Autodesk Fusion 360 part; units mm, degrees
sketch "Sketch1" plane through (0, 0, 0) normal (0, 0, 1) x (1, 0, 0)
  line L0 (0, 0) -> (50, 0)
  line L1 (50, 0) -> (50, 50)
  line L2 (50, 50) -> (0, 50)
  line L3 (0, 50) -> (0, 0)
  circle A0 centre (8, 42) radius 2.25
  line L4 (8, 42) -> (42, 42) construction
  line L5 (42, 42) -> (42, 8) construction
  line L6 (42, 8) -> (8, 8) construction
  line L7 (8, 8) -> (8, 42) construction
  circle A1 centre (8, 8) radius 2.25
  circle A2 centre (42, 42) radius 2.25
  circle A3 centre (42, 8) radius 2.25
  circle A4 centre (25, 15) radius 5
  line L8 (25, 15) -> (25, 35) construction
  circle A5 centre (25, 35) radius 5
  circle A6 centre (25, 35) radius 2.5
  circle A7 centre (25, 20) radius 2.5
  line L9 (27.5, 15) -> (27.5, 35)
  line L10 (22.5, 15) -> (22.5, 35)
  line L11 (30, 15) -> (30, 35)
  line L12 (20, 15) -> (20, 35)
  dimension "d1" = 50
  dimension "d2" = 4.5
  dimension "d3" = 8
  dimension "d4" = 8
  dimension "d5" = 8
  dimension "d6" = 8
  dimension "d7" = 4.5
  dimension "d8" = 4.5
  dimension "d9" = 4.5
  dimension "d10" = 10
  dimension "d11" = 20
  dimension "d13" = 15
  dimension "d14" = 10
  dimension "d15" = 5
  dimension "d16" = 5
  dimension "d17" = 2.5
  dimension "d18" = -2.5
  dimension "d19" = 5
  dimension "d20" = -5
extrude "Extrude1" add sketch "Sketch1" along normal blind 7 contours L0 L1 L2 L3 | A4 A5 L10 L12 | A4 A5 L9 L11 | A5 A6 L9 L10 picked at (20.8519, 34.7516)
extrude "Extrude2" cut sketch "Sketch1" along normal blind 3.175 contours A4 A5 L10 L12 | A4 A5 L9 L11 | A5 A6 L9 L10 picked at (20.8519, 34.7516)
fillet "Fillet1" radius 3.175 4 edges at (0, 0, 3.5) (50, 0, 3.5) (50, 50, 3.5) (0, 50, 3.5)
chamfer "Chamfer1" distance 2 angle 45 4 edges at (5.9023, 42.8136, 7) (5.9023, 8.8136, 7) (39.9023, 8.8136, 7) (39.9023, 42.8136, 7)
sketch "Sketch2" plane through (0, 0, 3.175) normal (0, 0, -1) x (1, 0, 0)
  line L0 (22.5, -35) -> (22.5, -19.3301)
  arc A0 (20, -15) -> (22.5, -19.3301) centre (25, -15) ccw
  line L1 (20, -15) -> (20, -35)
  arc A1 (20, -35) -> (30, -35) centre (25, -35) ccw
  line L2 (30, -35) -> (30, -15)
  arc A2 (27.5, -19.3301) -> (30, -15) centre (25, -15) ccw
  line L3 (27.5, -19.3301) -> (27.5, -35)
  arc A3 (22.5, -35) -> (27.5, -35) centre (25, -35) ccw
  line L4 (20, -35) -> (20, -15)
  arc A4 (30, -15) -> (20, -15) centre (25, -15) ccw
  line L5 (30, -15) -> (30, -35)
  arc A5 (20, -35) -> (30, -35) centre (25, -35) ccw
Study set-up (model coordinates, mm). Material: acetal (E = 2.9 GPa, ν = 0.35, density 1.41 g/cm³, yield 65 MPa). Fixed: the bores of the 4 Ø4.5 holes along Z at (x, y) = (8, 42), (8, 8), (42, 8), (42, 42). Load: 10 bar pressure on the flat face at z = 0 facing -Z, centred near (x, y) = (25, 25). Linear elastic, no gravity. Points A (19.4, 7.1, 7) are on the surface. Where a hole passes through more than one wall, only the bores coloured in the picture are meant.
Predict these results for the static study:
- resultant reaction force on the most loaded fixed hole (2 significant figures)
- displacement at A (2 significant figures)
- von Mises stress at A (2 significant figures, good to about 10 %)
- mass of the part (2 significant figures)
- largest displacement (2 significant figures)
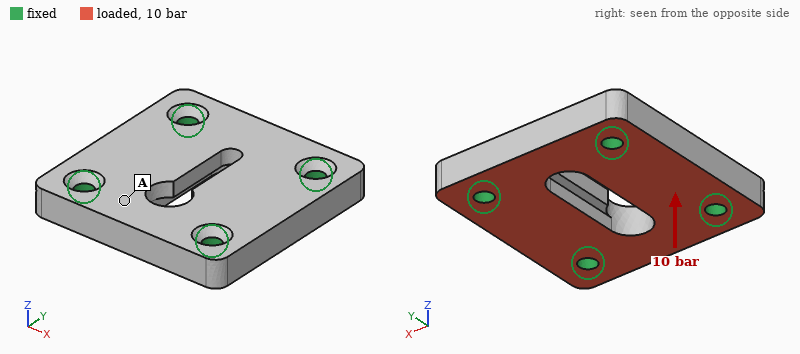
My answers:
540 N
0.073 mm
6.7 MPa
22 g
0.16 mm
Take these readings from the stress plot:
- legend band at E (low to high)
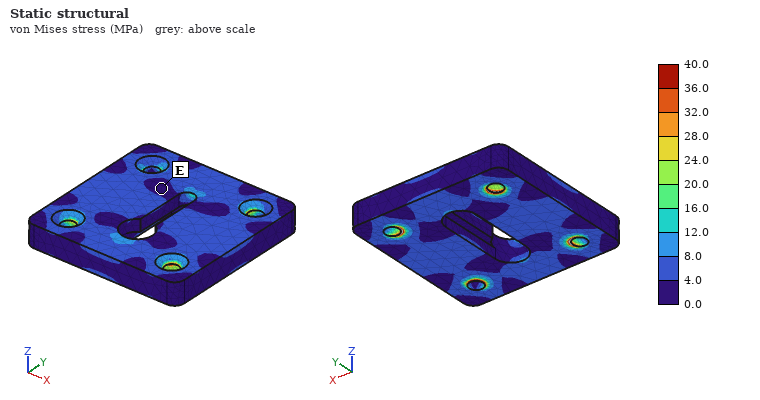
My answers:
0.0 to 4.0 MPa
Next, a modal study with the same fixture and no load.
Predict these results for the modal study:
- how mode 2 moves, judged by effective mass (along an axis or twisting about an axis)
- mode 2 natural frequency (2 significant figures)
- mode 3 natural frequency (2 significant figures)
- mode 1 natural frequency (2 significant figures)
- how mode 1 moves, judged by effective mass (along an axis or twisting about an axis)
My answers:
twisting about Y
6100 Hz
6400 Hz
5000 Hz
along Z
